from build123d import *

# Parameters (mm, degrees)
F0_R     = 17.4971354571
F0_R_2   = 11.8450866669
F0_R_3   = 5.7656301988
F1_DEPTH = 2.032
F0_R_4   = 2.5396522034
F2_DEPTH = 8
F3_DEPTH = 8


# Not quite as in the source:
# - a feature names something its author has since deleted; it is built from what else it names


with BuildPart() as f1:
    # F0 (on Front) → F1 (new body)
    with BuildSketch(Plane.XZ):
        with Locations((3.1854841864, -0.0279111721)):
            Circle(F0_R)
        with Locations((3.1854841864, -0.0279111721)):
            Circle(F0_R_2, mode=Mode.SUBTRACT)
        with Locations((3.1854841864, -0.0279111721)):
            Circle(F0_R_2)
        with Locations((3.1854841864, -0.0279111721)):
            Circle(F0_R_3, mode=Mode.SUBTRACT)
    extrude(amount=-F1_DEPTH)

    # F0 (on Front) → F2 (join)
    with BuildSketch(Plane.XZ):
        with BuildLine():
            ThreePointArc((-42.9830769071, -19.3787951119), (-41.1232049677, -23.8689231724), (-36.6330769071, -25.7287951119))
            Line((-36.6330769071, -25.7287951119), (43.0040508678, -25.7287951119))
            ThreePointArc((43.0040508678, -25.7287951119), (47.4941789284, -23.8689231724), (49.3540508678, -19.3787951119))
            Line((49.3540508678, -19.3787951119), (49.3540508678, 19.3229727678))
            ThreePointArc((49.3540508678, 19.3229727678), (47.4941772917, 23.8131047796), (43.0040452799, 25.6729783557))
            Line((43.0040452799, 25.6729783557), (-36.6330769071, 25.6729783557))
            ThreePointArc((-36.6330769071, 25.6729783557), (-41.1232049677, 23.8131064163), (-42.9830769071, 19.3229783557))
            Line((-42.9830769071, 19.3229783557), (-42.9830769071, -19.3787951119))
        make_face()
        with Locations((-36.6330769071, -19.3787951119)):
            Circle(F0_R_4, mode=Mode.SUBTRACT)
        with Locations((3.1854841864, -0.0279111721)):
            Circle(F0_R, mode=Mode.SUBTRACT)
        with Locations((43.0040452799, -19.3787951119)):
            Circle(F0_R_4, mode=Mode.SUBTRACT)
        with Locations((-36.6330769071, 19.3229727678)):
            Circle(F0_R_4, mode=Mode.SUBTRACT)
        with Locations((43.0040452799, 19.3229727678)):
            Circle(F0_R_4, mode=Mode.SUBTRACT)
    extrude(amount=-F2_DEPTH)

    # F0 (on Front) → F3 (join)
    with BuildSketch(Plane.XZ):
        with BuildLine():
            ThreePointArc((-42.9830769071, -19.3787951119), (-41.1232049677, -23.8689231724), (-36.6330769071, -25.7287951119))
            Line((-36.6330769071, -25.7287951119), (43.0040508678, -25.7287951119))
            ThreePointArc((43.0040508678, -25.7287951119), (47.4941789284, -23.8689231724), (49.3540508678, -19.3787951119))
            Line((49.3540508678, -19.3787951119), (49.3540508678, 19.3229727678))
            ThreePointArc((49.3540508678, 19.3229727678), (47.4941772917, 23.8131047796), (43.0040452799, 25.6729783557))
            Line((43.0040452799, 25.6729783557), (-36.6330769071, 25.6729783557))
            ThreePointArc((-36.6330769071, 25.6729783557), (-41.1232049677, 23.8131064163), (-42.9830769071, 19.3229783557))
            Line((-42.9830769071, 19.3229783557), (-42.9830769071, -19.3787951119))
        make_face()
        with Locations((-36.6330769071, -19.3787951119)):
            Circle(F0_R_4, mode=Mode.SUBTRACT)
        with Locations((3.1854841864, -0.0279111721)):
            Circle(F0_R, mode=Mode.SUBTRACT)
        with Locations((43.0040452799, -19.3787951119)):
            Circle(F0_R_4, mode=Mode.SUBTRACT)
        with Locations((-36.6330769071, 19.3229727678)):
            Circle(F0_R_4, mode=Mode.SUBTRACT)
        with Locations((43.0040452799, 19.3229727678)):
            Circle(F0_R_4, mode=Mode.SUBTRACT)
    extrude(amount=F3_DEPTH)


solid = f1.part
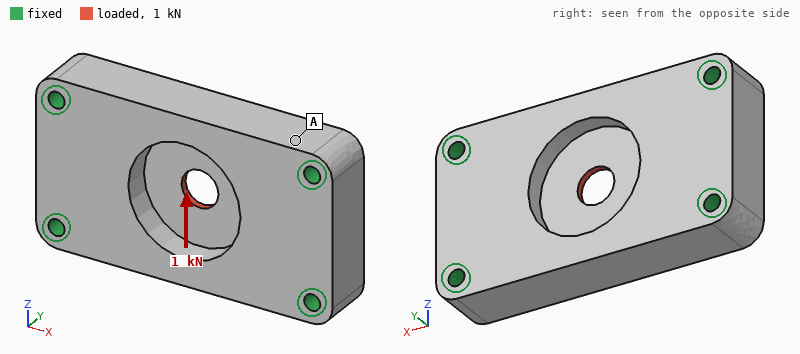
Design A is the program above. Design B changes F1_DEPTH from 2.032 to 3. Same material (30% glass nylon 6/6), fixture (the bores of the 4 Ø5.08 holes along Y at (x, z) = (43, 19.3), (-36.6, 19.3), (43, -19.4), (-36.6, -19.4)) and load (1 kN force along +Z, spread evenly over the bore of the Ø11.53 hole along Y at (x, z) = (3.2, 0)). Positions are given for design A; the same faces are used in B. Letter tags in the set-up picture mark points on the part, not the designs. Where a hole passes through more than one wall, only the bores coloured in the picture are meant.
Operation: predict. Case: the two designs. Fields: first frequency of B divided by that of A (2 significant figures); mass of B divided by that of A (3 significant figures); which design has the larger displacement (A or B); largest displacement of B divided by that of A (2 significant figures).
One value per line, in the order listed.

0.99
1.01
A
0.80
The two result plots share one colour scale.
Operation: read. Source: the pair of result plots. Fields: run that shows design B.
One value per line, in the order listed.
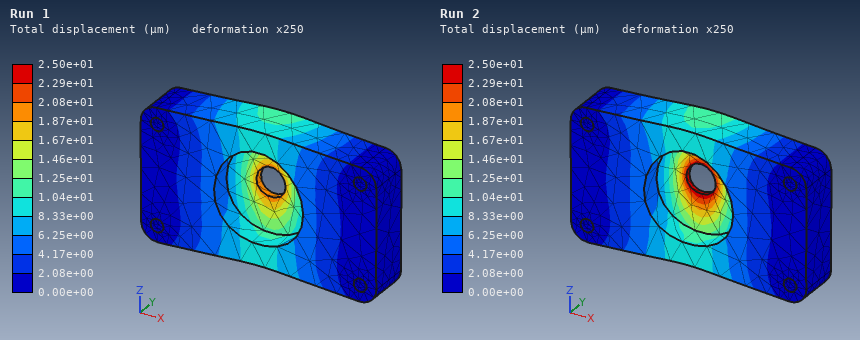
Run 1
